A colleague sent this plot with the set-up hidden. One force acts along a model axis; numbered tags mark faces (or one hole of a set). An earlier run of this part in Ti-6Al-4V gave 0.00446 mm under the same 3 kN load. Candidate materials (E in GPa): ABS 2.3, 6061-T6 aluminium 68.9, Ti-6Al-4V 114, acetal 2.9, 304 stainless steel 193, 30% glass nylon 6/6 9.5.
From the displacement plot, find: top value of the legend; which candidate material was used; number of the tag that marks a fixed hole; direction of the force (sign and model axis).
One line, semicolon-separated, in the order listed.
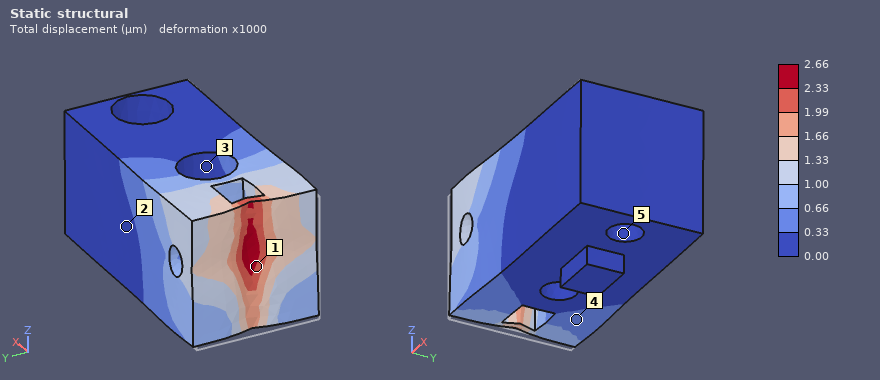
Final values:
2.66 µm; 304 stainless steel; 5; +X
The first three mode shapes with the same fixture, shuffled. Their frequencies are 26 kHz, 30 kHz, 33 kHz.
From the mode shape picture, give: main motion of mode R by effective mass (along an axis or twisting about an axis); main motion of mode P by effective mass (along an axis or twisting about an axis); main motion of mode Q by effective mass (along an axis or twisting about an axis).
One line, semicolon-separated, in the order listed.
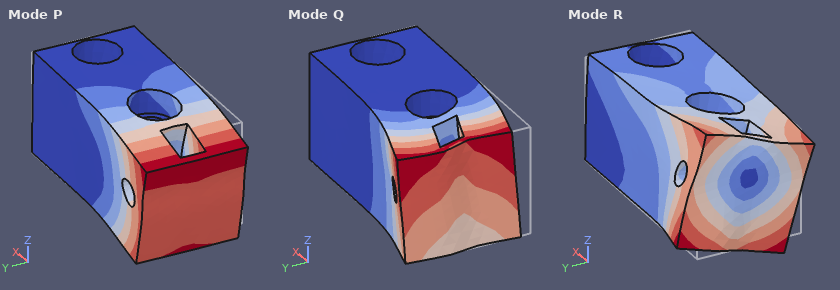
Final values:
twisting about X; along Z; along Y
